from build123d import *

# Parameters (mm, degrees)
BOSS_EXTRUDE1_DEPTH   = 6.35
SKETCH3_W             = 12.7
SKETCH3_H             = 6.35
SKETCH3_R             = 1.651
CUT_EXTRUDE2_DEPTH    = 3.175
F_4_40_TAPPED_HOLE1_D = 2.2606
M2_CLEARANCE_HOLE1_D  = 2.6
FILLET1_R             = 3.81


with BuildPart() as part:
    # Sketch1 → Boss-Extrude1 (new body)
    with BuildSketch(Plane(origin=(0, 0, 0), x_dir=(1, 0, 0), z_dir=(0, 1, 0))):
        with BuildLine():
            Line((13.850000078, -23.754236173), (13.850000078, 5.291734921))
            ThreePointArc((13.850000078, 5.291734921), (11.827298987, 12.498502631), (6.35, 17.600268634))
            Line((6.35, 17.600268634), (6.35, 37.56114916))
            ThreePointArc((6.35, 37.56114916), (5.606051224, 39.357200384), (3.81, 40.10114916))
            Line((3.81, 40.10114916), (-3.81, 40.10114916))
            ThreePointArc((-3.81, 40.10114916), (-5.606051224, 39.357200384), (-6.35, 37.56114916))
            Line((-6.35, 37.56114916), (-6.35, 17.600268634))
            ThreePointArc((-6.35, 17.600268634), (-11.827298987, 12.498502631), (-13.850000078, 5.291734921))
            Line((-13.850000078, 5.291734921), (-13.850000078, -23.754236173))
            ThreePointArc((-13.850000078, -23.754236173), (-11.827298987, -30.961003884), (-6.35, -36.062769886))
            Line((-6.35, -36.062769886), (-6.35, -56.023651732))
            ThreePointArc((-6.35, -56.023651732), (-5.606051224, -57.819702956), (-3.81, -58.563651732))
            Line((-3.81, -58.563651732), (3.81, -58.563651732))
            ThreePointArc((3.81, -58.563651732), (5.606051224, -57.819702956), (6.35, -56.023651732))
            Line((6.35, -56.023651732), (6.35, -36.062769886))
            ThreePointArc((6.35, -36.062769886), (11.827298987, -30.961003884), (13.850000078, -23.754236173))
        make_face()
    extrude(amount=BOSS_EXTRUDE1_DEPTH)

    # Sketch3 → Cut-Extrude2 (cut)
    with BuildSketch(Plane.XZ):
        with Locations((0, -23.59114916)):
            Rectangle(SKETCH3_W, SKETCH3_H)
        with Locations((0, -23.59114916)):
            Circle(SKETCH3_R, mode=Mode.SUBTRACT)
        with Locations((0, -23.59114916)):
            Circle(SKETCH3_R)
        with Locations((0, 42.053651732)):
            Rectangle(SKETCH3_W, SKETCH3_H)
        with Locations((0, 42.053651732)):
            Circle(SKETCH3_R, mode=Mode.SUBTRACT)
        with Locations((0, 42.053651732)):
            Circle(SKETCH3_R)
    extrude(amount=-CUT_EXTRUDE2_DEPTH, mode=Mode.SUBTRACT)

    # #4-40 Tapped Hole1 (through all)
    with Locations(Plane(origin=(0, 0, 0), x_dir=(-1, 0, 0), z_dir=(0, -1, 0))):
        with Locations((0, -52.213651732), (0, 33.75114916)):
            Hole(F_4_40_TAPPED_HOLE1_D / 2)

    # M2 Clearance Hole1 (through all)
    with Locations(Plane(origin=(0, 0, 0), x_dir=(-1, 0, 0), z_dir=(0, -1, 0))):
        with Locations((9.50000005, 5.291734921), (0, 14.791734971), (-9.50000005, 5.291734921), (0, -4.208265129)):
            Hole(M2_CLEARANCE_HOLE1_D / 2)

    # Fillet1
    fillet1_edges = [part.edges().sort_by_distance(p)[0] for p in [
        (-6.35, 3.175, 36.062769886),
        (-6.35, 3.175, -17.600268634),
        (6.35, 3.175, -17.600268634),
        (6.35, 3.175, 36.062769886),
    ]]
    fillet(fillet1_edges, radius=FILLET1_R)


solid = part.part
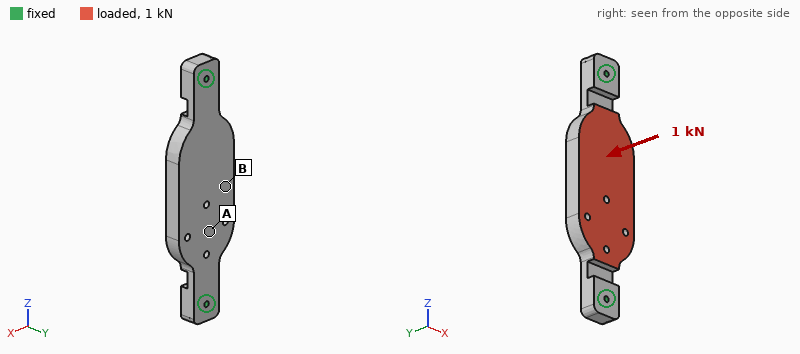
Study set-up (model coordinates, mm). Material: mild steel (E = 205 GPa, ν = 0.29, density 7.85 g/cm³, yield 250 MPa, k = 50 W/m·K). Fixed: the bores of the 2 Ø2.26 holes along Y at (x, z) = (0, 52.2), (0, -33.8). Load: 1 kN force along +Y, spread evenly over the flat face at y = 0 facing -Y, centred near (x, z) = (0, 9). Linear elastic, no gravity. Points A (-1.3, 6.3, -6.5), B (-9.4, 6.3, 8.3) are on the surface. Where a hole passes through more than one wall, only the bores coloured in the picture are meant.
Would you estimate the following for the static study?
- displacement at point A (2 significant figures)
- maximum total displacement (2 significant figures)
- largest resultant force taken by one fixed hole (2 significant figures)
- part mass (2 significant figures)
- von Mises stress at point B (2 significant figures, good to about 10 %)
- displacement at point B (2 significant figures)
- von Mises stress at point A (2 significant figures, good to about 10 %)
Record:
36 µm
46 µm
720 N
92 g
42 MPa
45 µm
34 MPa
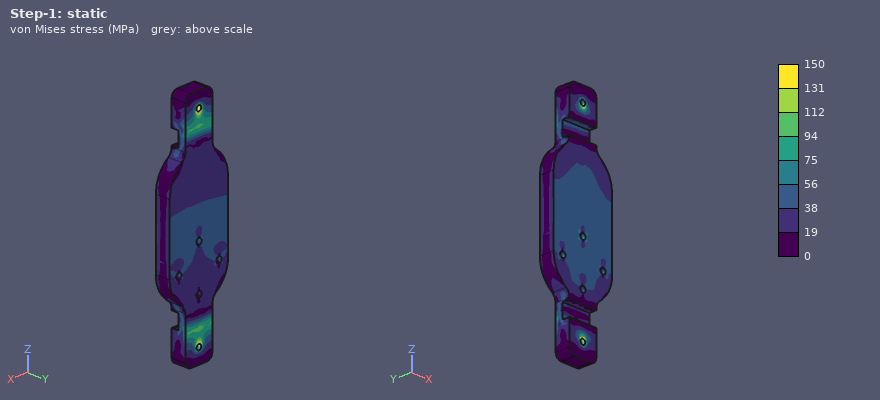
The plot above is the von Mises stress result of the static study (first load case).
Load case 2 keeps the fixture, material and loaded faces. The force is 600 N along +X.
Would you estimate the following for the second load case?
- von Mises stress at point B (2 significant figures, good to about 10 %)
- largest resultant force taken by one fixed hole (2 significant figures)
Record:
7.2 MPa
300 N
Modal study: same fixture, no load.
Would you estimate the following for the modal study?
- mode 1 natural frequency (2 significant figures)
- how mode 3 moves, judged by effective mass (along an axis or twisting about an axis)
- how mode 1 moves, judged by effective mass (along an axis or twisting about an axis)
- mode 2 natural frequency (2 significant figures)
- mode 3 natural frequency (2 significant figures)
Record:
3000 Hz
along X
along Y
3700 Hz
6200 Hz
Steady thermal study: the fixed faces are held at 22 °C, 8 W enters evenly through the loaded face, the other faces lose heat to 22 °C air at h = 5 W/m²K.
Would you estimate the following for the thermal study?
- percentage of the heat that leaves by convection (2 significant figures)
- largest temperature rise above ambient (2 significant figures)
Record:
5.4 %
33 K
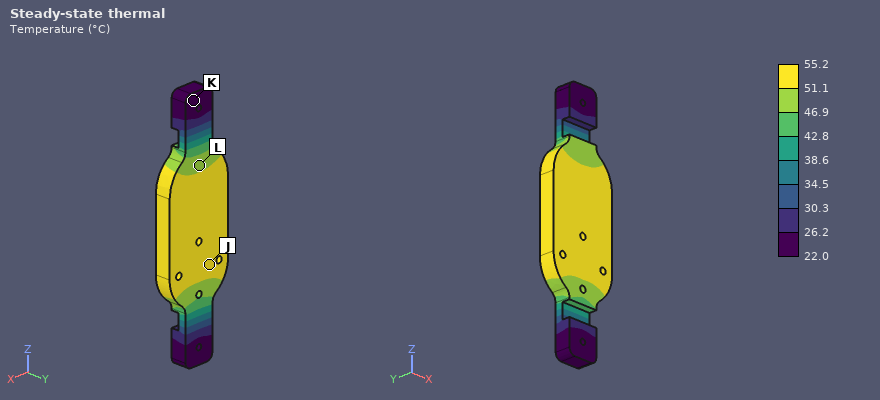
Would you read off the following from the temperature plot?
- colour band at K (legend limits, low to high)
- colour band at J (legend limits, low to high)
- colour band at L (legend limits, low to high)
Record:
22.0 to 26.2 °C
51.1 to 55.2 °C
46.9 to 51.1 °C
